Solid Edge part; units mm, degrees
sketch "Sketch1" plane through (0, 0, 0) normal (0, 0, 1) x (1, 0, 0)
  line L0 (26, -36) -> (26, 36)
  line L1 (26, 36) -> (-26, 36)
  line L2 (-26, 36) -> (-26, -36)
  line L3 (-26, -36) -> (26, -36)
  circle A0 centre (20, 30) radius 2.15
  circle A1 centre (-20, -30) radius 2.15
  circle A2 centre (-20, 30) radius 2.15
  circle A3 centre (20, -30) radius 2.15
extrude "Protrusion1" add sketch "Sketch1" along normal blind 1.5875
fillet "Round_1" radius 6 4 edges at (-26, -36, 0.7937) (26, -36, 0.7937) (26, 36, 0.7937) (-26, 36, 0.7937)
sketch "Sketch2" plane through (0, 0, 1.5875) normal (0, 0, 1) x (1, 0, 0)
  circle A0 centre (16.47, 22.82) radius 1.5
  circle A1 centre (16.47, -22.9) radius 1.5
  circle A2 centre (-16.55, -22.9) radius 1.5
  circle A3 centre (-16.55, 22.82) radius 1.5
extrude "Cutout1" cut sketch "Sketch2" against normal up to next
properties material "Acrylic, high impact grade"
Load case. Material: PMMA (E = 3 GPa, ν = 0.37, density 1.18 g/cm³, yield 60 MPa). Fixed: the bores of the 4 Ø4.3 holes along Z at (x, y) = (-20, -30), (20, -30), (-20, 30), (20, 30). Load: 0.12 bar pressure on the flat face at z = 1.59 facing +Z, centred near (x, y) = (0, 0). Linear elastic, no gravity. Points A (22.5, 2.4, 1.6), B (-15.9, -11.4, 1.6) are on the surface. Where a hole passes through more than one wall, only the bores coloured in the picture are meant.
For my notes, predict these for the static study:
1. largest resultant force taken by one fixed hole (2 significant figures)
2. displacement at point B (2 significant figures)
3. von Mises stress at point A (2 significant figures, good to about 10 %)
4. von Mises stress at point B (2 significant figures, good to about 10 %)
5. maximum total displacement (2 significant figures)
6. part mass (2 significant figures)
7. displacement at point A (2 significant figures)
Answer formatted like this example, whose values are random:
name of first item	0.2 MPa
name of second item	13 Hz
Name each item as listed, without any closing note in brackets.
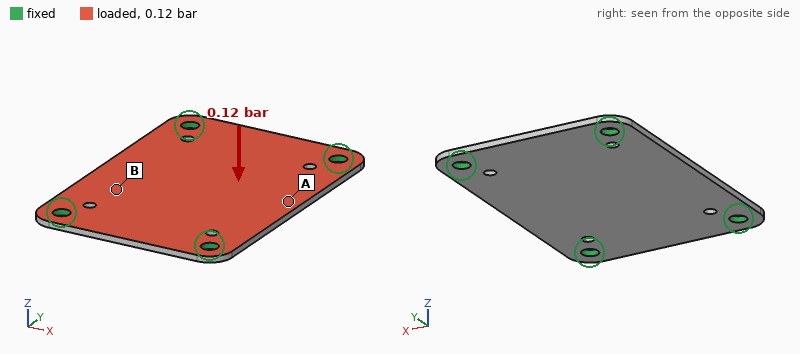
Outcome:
largest resultant force taken by one fixed hole	11 N
displacement at point B	0.33 mm
von Mises stress at point A	4.6 MPa
von Mises stress at point B	2.8 MPa
maximum total displacement	0.48 mm
part mass	6.8 g
displacement at point A	0.42 mm
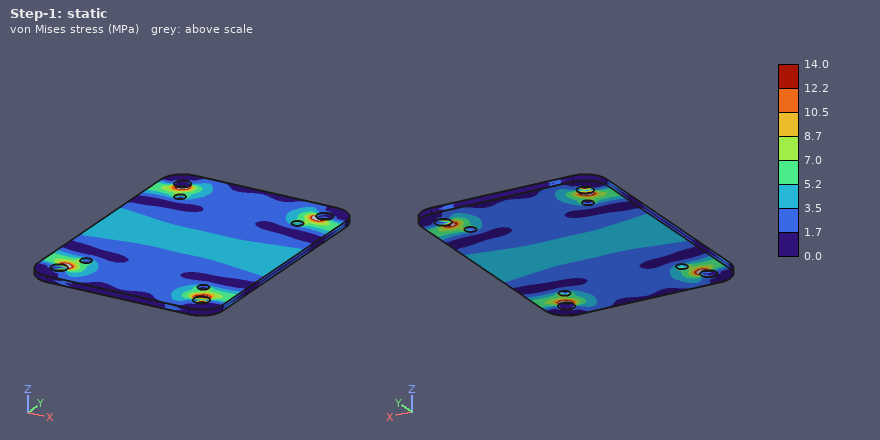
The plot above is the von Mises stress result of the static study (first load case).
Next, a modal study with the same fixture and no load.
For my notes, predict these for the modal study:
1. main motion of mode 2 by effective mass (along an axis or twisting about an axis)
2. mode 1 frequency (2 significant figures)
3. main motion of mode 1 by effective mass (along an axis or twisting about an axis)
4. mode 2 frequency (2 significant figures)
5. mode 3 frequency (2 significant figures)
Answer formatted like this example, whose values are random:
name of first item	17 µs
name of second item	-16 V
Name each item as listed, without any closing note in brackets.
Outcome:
main motion of mode 2 by effective mass	twisting about Y
mode 1 frequency	680 Hz
main motion of mode 1 by effective mass	along Z
mode 2 frequency	960 Hz
mode 3 frequency	1500 Hz
